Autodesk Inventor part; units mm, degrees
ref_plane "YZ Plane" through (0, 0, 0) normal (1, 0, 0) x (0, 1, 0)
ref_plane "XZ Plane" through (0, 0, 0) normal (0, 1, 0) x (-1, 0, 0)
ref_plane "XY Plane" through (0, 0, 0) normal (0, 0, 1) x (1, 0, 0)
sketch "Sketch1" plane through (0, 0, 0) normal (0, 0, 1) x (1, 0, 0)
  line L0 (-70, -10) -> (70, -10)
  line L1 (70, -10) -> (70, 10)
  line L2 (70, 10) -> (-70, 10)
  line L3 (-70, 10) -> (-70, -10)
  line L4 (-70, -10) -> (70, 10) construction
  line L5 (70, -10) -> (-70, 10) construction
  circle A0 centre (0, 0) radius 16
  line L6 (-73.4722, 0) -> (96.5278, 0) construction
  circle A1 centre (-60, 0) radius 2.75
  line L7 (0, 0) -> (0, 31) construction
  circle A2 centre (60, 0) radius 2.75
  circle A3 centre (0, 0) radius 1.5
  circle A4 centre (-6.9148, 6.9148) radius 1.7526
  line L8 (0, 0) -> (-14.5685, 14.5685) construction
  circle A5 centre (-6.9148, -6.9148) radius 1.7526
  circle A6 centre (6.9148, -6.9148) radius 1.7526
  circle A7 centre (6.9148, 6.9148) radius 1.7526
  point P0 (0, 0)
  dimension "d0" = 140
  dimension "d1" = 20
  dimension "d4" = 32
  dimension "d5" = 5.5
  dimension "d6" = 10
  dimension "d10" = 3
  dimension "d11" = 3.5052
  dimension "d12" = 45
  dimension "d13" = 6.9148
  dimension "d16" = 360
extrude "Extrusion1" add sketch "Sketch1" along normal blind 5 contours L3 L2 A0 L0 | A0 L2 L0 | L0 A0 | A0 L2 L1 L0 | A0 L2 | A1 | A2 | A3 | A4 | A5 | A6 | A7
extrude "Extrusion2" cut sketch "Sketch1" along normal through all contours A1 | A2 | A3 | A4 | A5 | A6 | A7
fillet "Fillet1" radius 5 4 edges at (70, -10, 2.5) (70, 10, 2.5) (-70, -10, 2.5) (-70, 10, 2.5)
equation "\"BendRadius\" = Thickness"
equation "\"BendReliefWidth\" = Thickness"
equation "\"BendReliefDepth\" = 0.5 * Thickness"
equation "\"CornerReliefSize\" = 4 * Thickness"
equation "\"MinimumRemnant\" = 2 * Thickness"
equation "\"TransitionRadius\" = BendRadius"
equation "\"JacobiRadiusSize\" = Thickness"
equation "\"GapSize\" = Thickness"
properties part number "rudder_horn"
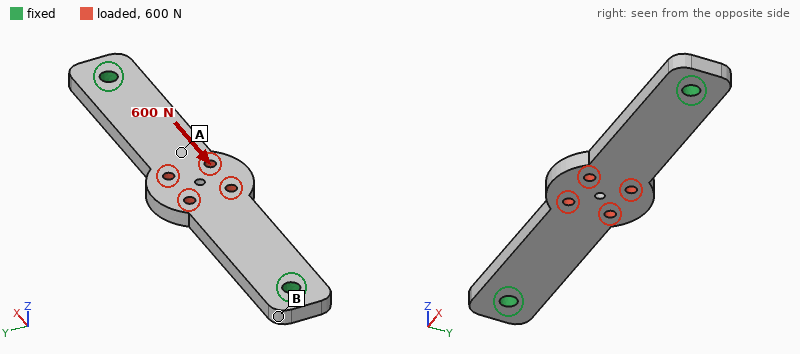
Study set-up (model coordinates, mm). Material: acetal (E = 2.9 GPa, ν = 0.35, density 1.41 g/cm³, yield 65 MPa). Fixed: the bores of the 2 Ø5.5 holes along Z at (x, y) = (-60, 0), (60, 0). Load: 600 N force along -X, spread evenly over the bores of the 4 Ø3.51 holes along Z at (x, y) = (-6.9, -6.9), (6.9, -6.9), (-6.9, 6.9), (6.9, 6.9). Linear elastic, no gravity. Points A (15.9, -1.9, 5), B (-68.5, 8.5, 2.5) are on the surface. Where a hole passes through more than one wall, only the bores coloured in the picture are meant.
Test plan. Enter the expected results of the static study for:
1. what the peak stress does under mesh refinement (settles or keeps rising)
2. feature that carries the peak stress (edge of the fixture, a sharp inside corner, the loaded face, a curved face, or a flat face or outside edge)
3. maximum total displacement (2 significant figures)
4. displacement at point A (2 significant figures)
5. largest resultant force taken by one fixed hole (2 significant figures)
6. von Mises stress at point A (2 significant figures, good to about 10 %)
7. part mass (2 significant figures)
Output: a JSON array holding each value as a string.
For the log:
["keeps rising", "edge of the fixture", "62 µm", "48 µm", "300 N", "2.6 MPa", "20 g"]
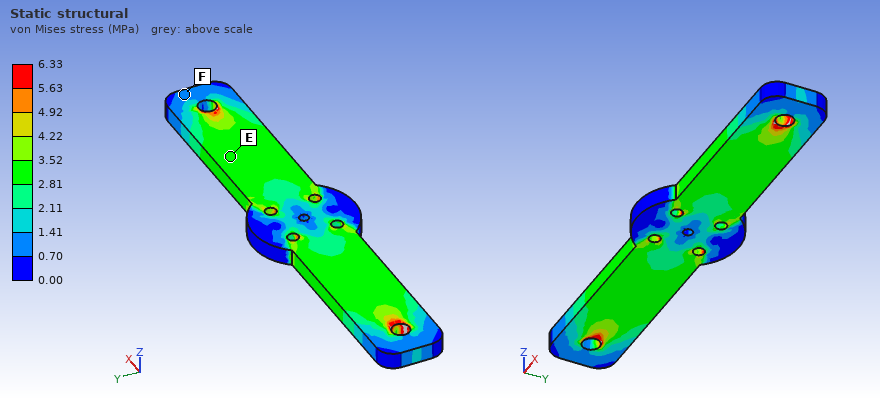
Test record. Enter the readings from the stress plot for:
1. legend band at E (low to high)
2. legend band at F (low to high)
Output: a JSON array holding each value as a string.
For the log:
["2.81 to 3.52 MPa", "0.70 to 1.41 MPa"]
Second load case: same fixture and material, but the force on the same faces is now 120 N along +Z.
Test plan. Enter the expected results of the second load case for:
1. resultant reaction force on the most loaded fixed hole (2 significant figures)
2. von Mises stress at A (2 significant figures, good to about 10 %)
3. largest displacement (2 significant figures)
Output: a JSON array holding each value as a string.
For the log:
["60 N", "10 MPa", "1.6 mm"]
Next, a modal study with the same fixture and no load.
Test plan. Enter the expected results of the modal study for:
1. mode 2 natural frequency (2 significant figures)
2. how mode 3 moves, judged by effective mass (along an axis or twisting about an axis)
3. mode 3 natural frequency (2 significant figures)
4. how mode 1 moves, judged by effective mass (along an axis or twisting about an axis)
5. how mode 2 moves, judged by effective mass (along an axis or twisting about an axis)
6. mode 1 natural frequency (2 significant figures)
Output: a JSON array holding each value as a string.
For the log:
["1300 Hz", "along Y", "1400 Hz", "along Z", "twisting about X", "490 Hz"]
